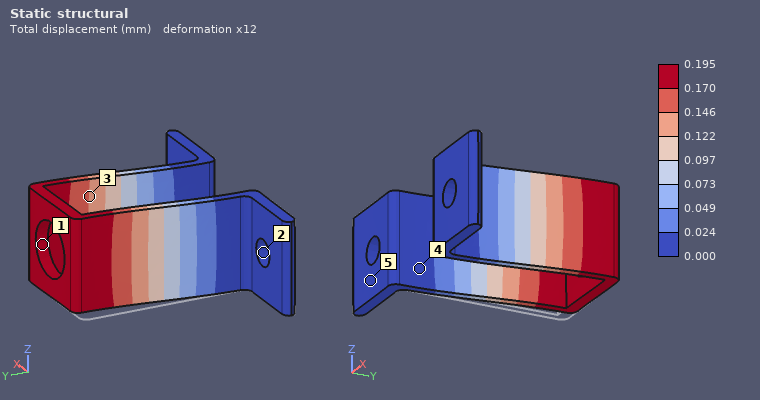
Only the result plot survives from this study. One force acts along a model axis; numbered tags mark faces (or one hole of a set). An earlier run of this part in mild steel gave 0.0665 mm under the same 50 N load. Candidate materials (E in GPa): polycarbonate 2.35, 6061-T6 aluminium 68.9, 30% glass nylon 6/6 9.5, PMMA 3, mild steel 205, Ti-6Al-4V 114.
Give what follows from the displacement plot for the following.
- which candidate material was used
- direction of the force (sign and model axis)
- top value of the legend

6061-T6 aluminium
+X
0.195 mm
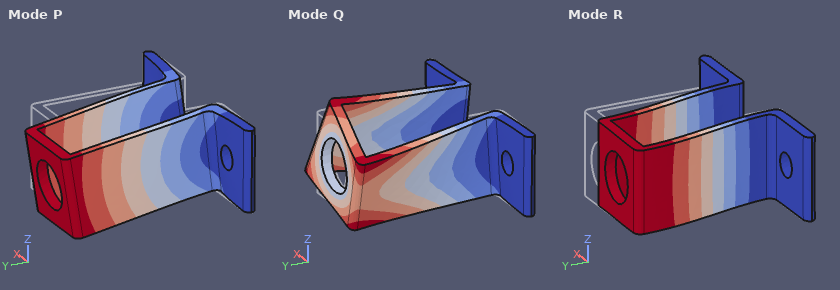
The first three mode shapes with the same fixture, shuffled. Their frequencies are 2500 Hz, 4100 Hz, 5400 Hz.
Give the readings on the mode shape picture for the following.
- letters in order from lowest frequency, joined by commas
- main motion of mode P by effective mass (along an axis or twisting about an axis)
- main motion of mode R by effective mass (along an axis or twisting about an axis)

R, P, Q
along Z
along X
